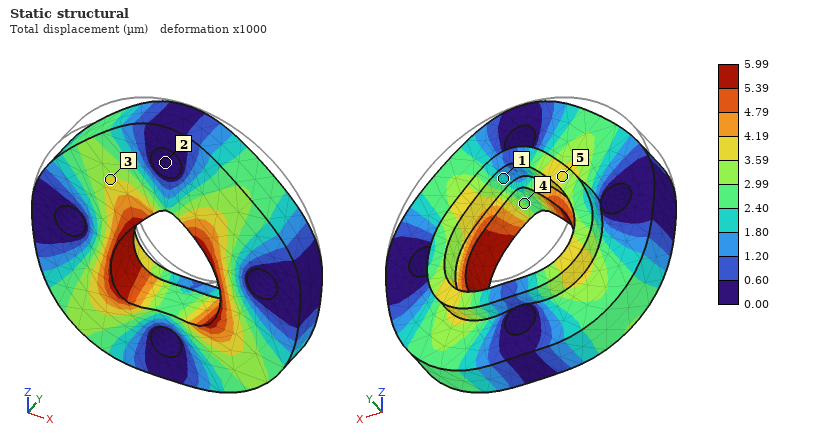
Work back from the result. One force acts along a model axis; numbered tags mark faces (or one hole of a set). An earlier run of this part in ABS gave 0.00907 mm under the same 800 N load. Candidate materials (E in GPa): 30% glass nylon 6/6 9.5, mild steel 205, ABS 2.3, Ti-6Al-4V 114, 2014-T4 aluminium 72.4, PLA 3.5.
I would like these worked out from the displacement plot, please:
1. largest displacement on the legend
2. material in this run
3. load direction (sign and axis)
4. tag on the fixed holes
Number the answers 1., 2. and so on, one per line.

1. 5.99 µm
2. PLA
3. -Z
4. 2
